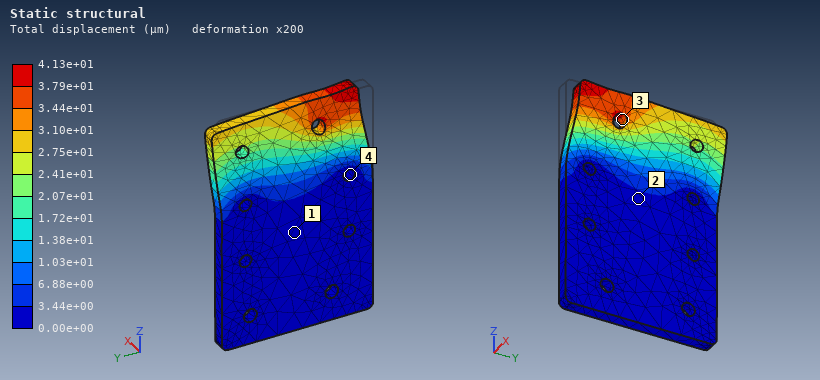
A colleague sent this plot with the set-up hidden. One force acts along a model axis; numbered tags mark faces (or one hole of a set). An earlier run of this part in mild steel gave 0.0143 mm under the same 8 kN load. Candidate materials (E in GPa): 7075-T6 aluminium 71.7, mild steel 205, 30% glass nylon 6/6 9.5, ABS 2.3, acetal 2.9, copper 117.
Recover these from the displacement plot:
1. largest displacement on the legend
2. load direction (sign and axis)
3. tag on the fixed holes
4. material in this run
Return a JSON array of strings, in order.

["4.13e+01 µm", "+Y", "4", "7075-T6 aluminium"]
